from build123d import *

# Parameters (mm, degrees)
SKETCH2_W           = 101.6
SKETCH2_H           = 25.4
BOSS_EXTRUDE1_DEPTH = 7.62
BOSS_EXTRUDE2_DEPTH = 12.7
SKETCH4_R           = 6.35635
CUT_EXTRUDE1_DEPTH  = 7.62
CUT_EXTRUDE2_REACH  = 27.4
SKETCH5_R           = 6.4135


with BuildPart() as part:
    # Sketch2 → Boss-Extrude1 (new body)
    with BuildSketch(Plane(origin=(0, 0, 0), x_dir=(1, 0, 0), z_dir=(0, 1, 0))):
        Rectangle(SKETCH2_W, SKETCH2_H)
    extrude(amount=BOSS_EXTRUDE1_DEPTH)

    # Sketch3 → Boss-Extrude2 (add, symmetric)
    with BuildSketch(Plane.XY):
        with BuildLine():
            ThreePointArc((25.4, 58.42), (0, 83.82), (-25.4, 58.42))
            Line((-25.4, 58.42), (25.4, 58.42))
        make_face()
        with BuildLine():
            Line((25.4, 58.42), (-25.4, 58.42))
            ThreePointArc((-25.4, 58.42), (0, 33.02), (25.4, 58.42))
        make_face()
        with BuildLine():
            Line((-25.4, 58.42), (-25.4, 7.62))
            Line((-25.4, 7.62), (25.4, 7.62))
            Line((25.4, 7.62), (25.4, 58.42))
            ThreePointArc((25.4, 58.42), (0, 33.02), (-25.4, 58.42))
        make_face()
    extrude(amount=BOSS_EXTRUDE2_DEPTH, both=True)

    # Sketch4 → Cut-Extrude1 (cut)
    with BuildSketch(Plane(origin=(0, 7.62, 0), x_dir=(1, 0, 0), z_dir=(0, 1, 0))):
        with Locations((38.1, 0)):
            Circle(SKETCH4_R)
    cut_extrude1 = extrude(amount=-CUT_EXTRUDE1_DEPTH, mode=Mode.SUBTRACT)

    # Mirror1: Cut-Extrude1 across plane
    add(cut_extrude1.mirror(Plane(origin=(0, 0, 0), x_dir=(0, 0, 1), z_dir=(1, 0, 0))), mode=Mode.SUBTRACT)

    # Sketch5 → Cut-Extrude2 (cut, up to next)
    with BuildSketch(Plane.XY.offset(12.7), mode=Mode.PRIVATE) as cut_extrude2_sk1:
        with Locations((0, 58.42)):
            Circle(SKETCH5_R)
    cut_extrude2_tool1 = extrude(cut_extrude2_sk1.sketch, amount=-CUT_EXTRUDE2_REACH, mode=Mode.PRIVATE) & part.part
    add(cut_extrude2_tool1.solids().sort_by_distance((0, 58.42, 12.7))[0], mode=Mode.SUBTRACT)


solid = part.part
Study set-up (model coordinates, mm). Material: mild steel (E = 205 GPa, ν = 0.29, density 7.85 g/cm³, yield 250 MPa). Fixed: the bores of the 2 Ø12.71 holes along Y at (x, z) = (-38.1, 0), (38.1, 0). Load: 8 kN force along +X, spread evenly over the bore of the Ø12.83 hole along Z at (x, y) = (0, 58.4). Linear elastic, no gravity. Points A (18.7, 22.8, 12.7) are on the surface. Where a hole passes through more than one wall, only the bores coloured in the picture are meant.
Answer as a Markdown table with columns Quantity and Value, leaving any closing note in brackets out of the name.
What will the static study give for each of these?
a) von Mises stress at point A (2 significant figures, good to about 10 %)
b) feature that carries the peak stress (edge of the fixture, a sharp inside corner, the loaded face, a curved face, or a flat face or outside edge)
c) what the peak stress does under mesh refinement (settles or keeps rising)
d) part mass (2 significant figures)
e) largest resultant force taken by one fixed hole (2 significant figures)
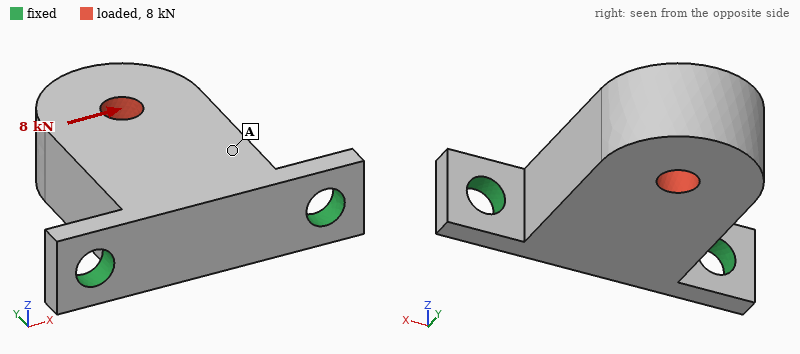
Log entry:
| Quantity | Value |
|---|---|
| von Mises stress at point A | 23 MPa |
| feature that carries the peak stress | edge of the fixture |
| what the peak stress does under mesh refinement | keeps rising |
| part mass | 830 g |
| largest resultant force taken by one fixed hole | 8.6 kN |
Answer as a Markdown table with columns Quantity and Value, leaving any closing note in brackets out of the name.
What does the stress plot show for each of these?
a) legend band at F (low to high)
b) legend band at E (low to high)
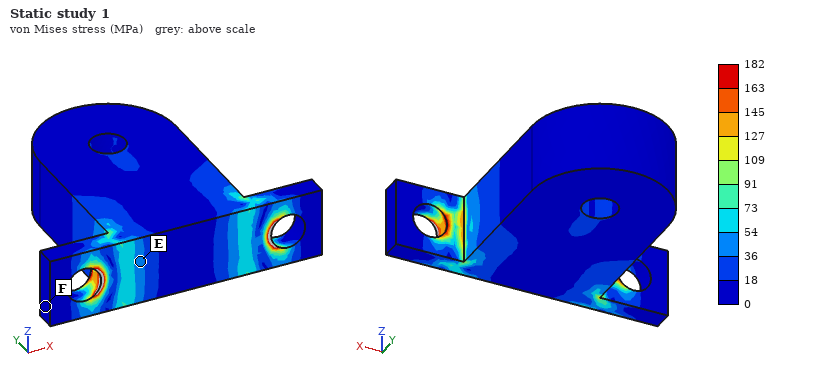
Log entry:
| Quantity | Value |
|---|---|
| legend band at F | 0 to 18 MPa |
| legend band at E | 36 to 54 MPa |
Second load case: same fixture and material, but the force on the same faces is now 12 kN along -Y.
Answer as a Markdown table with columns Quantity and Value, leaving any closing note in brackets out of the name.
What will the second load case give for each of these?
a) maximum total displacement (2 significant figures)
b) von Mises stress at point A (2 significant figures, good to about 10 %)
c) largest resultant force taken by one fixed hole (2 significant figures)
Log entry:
| Quantity | Value |
|---|---|
| maximum total displacement | 14 µm |
| von Mises stress at point A | 17 MPa |
| largest resultant force taken by one fixed hole | 6.6 kN |
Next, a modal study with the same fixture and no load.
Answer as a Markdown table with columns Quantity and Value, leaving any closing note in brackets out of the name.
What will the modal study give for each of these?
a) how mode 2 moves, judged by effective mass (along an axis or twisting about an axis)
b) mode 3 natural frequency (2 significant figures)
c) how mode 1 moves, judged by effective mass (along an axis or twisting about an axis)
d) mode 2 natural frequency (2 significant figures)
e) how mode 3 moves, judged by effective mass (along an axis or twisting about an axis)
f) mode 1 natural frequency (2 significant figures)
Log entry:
| Quantity | Value |
|---|---|
| how mode 2 moves, judged by effective mass | along X |
| mode 3 natural frequency | 5700 Hz |
| how mode 1 moves, judged by effective mass | along Z |
| mode 2 natural frequency | 3500 Hz |
| how mode 3 moves, judged by effective mass | along Y |
| mode 1 natural frequency | 1100 Hz |
